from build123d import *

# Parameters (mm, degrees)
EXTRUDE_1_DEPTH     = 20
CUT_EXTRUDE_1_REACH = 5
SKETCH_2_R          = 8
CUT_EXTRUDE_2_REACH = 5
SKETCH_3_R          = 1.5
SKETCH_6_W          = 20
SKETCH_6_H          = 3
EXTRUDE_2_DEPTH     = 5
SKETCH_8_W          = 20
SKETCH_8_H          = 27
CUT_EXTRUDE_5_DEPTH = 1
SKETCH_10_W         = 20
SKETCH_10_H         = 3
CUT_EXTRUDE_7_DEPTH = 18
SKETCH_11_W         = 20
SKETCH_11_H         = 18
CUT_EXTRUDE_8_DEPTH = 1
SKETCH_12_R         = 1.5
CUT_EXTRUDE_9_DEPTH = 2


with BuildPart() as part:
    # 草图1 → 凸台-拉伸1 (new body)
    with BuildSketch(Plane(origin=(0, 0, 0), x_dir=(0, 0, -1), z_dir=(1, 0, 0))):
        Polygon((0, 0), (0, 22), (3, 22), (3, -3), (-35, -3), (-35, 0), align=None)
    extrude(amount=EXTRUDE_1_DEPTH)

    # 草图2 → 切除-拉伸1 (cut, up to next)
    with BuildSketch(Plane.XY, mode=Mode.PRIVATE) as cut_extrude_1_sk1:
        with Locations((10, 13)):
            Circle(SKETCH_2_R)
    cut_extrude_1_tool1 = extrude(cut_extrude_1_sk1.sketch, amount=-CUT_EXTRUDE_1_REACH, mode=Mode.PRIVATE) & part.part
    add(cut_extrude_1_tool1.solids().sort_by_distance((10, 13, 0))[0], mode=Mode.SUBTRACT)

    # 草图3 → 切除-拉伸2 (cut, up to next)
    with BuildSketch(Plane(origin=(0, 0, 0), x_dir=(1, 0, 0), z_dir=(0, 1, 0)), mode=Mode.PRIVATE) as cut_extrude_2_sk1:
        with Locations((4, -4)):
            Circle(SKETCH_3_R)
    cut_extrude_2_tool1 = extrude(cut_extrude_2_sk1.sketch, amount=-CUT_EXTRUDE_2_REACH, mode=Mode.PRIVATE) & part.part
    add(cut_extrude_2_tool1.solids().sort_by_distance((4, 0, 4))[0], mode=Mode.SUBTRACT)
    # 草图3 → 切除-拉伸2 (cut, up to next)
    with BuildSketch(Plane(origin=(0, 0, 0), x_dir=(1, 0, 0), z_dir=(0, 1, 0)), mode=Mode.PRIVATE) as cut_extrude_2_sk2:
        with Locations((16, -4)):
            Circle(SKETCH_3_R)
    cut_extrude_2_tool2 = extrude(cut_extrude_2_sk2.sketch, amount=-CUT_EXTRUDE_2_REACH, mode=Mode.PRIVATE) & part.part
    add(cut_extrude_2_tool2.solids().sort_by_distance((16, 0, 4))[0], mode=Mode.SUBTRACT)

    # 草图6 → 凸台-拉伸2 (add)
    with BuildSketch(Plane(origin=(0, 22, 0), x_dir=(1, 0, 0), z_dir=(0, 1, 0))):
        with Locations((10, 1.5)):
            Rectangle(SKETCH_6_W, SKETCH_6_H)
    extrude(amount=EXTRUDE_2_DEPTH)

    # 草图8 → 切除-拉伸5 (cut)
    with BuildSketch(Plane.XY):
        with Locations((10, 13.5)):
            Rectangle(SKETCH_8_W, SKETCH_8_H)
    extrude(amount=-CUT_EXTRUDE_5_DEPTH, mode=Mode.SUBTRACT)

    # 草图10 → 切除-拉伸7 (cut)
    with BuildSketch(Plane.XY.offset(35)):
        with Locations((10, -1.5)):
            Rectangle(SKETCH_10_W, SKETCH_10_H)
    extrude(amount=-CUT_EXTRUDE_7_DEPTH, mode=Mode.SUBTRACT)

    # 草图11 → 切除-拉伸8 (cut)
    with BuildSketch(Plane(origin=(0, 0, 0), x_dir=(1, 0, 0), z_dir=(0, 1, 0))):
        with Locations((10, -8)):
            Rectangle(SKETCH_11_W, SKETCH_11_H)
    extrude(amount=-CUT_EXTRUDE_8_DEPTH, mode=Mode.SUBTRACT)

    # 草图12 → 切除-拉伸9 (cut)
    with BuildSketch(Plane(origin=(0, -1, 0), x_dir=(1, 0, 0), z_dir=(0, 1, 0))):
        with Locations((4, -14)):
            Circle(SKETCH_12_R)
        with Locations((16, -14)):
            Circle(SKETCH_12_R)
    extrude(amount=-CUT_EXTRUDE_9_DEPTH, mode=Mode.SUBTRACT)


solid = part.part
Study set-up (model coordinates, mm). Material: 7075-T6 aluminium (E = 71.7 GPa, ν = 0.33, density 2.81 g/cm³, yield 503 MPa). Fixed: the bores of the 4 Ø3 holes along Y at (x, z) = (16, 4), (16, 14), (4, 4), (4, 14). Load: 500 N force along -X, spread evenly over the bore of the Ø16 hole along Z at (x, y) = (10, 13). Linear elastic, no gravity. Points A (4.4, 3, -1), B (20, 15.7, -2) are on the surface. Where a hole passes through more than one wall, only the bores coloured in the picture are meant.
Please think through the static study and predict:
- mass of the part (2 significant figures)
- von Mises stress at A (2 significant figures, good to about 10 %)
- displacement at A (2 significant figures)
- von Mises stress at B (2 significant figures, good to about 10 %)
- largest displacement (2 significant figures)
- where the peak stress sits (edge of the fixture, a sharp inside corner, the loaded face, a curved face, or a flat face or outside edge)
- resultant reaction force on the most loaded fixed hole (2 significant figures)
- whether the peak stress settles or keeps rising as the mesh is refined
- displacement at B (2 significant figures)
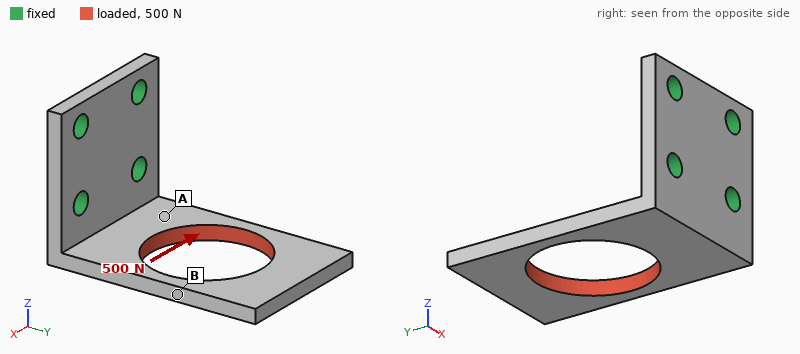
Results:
4.1 g
58 MPa
0.055 mm
150 MPa
0.33 mm
edge of the fixture
640 N
keeps rising
0.24 mm
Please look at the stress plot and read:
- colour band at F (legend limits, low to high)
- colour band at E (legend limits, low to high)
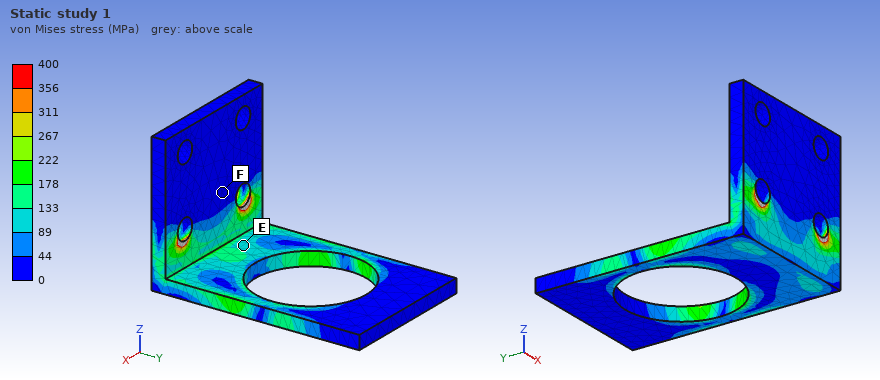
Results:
0 to 44 MPa
89 to 133 MPa
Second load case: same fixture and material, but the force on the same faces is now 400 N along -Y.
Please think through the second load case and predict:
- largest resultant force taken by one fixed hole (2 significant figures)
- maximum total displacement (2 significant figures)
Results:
210 N
0.17 mm
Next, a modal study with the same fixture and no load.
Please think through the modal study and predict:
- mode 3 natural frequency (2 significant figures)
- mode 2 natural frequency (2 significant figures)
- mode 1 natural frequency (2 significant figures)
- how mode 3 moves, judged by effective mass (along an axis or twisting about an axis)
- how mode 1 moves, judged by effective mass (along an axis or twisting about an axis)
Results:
5300 Hz
4200 Hz
1400 Hz
along X
along Z
